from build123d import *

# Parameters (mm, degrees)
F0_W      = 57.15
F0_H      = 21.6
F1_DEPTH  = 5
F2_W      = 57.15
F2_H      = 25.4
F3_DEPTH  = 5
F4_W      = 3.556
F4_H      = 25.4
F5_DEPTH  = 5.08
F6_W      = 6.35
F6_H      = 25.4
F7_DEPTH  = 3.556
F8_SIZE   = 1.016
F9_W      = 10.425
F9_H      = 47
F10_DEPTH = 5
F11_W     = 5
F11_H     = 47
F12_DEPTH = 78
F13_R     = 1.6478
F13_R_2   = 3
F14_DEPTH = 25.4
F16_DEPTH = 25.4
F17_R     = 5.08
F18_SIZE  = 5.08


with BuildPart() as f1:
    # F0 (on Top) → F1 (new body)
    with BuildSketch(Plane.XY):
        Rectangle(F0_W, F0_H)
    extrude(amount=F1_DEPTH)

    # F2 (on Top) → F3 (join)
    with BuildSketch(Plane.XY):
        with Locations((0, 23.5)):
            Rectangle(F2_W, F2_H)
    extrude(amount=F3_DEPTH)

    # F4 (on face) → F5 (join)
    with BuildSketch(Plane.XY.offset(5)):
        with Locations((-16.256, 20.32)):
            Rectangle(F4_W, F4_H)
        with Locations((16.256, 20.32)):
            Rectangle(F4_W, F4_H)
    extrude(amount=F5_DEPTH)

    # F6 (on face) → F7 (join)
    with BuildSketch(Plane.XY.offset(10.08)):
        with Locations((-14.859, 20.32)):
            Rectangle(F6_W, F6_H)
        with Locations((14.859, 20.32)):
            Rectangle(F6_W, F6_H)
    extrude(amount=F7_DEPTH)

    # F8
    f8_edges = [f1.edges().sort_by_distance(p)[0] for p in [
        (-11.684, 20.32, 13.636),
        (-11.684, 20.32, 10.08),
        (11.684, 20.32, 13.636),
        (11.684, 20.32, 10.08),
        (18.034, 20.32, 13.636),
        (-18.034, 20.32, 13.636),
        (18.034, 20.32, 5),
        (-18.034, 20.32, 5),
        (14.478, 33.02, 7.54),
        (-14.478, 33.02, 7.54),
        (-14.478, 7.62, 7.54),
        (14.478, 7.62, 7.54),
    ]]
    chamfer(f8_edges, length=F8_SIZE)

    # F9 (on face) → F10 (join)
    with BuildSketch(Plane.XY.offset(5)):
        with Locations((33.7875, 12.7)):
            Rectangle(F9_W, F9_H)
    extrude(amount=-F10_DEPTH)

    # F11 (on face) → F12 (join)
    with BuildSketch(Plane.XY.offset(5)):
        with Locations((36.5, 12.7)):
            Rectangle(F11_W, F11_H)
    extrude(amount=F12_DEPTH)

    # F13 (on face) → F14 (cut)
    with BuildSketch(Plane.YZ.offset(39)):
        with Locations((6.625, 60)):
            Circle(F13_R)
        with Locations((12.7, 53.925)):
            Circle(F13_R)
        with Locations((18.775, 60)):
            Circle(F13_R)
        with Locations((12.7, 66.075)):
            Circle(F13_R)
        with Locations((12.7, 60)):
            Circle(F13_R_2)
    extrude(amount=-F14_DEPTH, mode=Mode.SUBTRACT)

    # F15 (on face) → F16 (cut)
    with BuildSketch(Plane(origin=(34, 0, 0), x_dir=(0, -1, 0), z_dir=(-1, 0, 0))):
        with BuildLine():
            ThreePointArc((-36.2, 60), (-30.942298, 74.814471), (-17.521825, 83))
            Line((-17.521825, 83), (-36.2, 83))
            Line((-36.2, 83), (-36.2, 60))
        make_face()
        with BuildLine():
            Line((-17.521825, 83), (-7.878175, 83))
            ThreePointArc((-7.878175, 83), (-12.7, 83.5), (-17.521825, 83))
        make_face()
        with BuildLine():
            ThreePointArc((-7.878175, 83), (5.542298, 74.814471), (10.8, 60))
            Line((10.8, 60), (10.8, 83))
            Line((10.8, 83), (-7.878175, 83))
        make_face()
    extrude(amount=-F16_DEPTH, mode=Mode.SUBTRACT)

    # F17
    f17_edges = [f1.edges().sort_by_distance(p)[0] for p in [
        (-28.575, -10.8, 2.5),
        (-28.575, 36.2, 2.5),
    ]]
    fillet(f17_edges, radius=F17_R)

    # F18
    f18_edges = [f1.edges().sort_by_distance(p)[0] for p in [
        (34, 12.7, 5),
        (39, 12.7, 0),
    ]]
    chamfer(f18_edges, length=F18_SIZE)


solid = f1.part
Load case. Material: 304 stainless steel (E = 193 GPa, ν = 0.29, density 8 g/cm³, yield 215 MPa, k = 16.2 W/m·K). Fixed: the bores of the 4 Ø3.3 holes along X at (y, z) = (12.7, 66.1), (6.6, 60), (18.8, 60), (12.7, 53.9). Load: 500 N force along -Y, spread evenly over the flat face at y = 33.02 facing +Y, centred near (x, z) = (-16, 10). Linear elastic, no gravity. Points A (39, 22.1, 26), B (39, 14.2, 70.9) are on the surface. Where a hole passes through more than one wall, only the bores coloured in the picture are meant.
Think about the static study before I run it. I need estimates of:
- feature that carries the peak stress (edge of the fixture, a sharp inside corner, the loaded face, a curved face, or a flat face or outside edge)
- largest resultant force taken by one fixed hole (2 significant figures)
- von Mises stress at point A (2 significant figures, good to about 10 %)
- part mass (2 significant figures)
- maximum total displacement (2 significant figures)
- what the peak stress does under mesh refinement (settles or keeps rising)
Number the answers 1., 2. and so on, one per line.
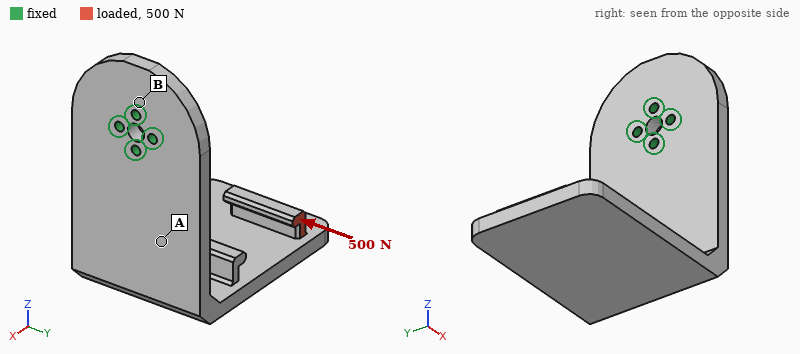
1. edge of the fixture
2. 1.2 kN
3. 100 MPa
4. 280 g
5. 0.57 mm
6. keeps rising
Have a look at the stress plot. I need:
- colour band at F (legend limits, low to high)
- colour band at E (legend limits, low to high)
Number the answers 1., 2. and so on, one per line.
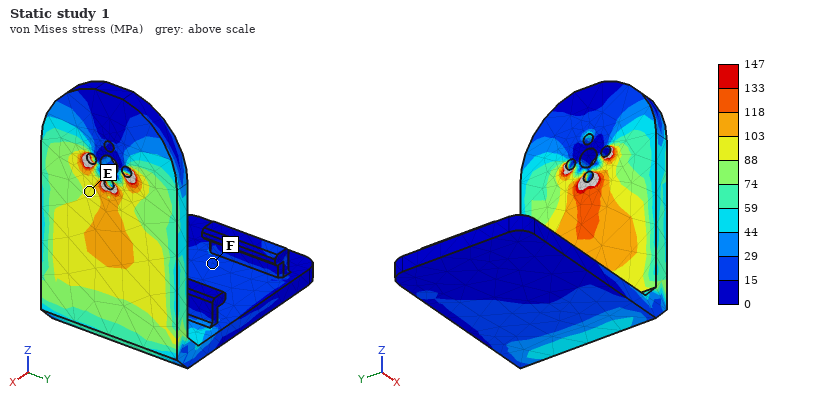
1. 15 to 29 MPa
2. 88 to 103 MPa
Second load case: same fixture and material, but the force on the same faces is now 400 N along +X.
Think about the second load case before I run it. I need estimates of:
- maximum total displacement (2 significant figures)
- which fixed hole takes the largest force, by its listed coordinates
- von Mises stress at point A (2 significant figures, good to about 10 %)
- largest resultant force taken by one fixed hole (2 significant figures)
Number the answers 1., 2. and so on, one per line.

1. 0.37 mm
2. (12.7, 53.9)
3. 41 MPa
4. 1.1 kN
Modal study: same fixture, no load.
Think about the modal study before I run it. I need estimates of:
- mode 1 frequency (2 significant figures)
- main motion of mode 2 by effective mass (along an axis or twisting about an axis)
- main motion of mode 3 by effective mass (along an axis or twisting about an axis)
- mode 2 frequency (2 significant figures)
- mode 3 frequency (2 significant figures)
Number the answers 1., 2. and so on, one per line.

1. 370 Hz
2. along Y
3. along X
4. 590 Hz
5. 1100 Hz
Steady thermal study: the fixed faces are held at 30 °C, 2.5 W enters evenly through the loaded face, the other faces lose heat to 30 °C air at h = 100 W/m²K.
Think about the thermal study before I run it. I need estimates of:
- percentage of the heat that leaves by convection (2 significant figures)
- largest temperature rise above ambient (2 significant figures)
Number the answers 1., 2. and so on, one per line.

1. 100 %
2. 38 K
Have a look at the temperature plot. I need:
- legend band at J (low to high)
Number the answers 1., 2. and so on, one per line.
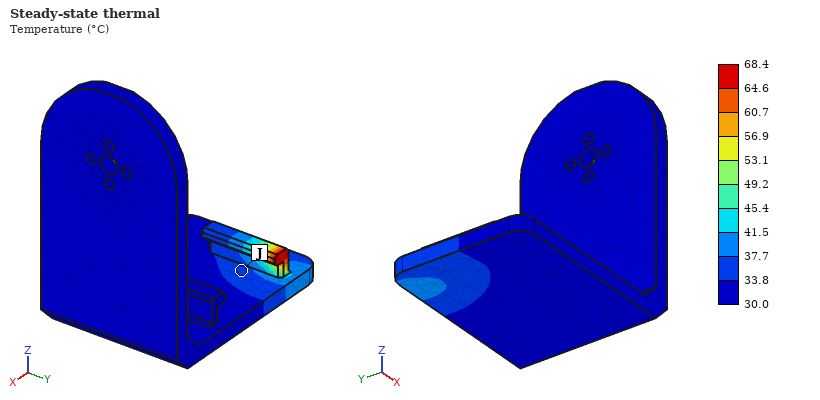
1. 33.8 to 37.7 °C
